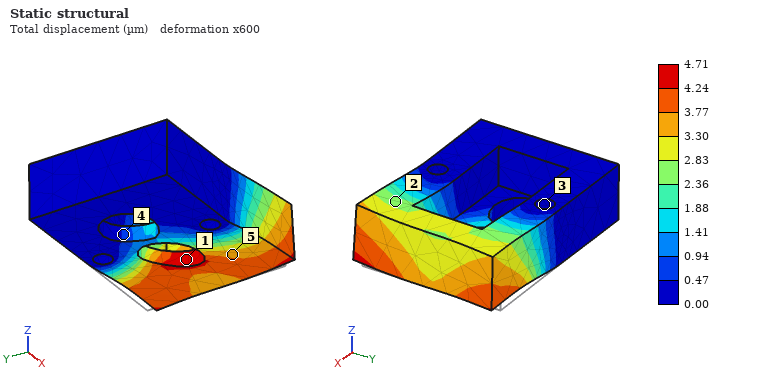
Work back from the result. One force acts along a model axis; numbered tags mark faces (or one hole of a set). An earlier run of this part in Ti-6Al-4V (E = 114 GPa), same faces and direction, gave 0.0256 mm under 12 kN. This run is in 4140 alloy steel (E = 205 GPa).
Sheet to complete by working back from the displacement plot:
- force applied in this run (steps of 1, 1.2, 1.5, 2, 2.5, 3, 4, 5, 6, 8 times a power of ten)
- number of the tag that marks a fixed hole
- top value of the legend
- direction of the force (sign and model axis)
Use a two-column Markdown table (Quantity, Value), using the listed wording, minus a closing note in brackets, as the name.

| Quantity | Value |
|---|---|
| force applied in this run | 4 kN |
| number of the tag that marks a fixed hole | 3 |
| top value of the legend | 4.71 µm |
| direction of the force | -Y |
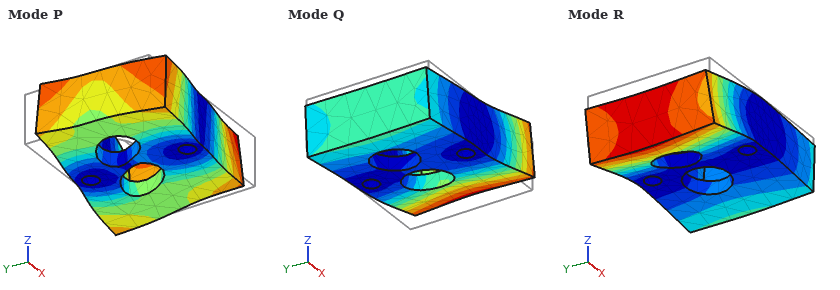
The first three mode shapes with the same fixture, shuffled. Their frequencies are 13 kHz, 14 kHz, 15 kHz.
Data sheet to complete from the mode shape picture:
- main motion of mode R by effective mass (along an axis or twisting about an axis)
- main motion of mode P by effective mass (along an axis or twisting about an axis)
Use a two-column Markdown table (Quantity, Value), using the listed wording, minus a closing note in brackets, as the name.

| Quantity | Value |
|---|---|
| main motion of mode R by effective mass | along Z |
| main motion of mode P by effective mass | twisting about Z |
